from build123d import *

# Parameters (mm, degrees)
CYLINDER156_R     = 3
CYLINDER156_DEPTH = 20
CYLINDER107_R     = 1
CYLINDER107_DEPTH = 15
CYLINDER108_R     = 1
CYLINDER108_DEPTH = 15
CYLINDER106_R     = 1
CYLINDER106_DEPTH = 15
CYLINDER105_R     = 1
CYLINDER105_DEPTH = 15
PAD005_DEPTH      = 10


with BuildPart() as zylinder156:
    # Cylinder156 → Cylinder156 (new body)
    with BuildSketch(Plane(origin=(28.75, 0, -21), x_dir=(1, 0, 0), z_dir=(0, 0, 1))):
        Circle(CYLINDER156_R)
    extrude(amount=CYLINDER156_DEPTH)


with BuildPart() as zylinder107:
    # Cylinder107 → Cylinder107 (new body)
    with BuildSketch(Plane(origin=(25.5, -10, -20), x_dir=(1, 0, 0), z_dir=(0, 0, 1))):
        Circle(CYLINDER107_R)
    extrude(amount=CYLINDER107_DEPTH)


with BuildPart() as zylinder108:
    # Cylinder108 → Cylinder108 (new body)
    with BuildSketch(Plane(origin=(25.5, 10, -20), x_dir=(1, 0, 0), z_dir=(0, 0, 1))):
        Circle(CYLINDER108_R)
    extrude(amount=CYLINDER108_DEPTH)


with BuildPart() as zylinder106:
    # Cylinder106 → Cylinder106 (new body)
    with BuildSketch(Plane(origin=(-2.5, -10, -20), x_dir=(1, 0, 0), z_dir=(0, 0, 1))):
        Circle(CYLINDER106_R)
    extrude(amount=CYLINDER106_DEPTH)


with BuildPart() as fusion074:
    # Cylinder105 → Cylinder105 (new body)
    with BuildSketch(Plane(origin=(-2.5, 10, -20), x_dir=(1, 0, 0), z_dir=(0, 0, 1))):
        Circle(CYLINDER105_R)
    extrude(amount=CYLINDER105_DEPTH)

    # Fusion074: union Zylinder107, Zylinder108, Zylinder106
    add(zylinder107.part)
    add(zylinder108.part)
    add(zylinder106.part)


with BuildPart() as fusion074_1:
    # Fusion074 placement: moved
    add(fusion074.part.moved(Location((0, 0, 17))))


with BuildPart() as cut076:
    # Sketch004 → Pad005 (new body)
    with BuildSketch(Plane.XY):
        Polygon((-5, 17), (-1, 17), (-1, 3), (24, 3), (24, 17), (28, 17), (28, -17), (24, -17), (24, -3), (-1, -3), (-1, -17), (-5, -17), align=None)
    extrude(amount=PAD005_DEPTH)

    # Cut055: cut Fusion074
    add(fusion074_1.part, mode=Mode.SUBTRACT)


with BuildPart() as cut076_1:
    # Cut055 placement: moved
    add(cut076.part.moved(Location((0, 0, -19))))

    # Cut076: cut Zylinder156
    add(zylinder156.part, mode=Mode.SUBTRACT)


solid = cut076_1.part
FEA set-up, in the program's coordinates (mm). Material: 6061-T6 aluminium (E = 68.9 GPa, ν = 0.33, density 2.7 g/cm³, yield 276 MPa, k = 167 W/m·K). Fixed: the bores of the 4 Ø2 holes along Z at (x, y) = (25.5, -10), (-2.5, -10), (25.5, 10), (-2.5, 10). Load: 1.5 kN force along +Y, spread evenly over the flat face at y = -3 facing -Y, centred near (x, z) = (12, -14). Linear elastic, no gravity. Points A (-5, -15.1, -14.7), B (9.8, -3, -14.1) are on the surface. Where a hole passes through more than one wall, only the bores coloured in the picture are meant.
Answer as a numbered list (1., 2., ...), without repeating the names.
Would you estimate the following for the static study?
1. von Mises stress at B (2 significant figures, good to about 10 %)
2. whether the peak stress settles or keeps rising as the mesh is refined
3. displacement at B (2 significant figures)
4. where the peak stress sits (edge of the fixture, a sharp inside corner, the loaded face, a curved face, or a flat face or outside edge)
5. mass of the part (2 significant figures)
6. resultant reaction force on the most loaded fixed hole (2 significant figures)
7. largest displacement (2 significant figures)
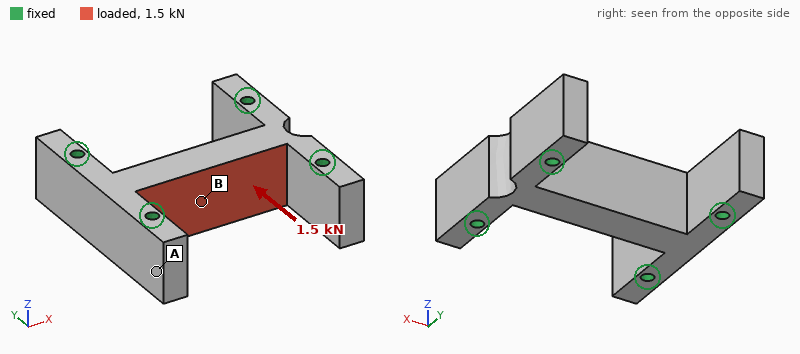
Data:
1. 37 MPa
2. keeps rising
3. 16 µm
4. a sharp inside corner
5. 11 g
6. 460 N
7. 17 µm
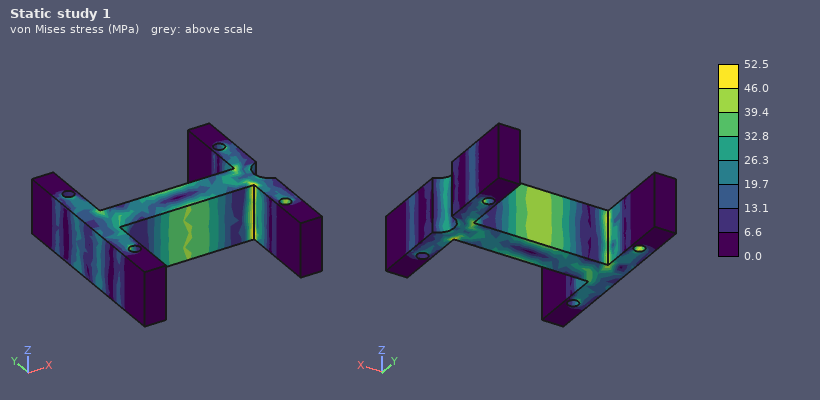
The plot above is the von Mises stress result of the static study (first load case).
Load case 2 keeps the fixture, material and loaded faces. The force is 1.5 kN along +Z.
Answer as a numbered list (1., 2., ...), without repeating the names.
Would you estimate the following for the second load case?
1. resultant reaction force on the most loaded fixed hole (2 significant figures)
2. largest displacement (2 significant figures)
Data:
1. 500 N
2. 25 µm
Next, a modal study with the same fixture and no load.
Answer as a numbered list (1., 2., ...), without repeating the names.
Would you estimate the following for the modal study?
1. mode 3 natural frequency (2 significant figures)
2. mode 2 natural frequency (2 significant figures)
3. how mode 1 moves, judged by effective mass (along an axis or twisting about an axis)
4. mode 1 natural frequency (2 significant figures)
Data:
1. 26 kHz
2. 25 kHz
3. along Z
4. 24 kHz
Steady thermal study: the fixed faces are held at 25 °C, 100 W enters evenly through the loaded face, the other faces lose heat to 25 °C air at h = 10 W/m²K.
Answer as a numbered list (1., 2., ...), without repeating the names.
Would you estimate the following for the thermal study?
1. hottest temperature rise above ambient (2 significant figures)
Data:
1. 69 K
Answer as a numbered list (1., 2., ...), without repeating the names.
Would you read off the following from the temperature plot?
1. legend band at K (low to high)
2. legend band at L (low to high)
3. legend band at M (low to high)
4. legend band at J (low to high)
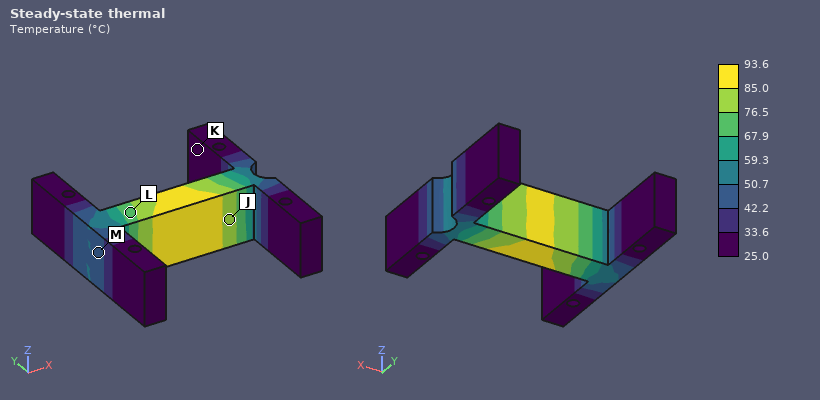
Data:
1. 25.0 to 33.6 °C
2. 67.9 to 76.5 °C
3. 42.2 to 50.7 °C
4. 76.5 to 85.0 °C
